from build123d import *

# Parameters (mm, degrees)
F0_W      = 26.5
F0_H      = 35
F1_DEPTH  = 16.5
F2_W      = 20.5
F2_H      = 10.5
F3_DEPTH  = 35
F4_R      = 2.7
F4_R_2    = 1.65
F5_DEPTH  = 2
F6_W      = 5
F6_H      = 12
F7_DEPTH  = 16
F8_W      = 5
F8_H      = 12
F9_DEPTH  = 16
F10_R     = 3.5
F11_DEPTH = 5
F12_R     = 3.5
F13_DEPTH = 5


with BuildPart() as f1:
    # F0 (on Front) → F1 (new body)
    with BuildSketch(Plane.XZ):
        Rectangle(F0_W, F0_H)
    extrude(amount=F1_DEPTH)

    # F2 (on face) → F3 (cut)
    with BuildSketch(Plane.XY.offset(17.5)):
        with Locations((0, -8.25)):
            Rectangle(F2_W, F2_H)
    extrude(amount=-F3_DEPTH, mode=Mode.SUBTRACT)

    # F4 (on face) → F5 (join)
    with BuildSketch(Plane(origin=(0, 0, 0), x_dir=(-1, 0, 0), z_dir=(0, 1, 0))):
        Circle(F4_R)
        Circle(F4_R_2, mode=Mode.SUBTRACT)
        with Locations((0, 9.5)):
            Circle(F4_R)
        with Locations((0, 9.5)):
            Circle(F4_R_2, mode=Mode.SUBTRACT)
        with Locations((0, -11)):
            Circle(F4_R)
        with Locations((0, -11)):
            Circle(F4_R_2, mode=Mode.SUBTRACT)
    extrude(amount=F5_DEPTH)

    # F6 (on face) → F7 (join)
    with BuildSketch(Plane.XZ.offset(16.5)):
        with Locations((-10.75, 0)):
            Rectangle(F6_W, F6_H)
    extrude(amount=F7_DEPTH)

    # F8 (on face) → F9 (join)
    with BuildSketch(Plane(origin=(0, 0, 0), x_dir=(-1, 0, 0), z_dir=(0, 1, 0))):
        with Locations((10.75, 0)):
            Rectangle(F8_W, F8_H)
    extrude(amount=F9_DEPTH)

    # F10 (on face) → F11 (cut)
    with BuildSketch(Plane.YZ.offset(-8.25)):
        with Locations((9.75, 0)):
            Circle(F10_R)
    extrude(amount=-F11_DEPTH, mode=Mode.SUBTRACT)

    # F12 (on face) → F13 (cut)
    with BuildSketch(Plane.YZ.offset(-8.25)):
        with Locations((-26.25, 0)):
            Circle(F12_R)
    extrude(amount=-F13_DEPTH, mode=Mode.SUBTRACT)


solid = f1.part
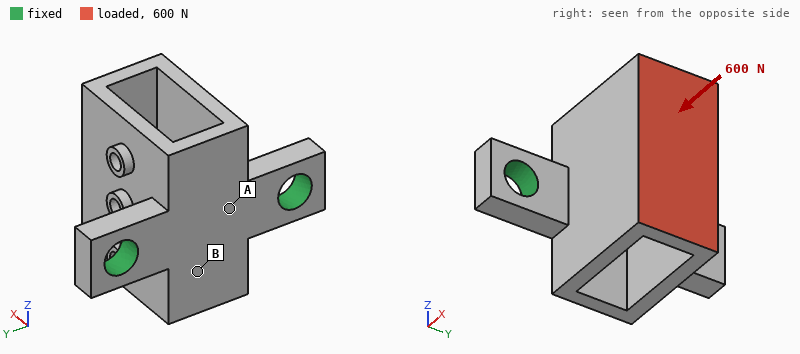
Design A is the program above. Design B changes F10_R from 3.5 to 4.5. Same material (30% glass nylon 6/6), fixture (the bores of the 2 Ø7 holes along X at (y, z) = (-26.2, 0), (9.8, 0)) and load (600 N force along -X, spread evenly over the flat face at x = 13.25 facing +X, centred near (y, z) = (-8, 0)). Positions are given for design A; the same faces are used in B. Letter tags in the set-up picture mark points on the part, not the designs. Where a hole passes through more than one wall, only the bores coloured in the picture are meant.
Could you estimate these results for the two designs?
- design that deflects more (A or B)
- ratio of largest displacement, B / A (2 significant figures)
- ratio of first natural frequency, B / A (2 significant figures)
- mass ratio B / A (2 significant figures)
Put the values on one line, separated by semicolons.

A; 0.92; 1.0; 0.99
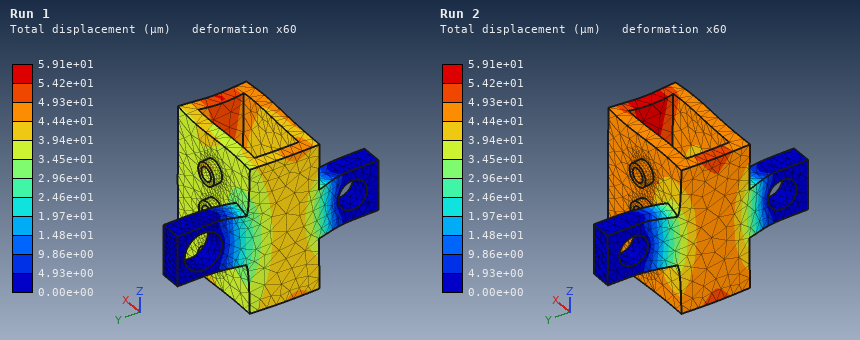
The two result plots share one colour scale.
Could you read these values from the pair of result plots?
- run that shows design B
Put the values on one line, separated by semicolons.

Run 1
